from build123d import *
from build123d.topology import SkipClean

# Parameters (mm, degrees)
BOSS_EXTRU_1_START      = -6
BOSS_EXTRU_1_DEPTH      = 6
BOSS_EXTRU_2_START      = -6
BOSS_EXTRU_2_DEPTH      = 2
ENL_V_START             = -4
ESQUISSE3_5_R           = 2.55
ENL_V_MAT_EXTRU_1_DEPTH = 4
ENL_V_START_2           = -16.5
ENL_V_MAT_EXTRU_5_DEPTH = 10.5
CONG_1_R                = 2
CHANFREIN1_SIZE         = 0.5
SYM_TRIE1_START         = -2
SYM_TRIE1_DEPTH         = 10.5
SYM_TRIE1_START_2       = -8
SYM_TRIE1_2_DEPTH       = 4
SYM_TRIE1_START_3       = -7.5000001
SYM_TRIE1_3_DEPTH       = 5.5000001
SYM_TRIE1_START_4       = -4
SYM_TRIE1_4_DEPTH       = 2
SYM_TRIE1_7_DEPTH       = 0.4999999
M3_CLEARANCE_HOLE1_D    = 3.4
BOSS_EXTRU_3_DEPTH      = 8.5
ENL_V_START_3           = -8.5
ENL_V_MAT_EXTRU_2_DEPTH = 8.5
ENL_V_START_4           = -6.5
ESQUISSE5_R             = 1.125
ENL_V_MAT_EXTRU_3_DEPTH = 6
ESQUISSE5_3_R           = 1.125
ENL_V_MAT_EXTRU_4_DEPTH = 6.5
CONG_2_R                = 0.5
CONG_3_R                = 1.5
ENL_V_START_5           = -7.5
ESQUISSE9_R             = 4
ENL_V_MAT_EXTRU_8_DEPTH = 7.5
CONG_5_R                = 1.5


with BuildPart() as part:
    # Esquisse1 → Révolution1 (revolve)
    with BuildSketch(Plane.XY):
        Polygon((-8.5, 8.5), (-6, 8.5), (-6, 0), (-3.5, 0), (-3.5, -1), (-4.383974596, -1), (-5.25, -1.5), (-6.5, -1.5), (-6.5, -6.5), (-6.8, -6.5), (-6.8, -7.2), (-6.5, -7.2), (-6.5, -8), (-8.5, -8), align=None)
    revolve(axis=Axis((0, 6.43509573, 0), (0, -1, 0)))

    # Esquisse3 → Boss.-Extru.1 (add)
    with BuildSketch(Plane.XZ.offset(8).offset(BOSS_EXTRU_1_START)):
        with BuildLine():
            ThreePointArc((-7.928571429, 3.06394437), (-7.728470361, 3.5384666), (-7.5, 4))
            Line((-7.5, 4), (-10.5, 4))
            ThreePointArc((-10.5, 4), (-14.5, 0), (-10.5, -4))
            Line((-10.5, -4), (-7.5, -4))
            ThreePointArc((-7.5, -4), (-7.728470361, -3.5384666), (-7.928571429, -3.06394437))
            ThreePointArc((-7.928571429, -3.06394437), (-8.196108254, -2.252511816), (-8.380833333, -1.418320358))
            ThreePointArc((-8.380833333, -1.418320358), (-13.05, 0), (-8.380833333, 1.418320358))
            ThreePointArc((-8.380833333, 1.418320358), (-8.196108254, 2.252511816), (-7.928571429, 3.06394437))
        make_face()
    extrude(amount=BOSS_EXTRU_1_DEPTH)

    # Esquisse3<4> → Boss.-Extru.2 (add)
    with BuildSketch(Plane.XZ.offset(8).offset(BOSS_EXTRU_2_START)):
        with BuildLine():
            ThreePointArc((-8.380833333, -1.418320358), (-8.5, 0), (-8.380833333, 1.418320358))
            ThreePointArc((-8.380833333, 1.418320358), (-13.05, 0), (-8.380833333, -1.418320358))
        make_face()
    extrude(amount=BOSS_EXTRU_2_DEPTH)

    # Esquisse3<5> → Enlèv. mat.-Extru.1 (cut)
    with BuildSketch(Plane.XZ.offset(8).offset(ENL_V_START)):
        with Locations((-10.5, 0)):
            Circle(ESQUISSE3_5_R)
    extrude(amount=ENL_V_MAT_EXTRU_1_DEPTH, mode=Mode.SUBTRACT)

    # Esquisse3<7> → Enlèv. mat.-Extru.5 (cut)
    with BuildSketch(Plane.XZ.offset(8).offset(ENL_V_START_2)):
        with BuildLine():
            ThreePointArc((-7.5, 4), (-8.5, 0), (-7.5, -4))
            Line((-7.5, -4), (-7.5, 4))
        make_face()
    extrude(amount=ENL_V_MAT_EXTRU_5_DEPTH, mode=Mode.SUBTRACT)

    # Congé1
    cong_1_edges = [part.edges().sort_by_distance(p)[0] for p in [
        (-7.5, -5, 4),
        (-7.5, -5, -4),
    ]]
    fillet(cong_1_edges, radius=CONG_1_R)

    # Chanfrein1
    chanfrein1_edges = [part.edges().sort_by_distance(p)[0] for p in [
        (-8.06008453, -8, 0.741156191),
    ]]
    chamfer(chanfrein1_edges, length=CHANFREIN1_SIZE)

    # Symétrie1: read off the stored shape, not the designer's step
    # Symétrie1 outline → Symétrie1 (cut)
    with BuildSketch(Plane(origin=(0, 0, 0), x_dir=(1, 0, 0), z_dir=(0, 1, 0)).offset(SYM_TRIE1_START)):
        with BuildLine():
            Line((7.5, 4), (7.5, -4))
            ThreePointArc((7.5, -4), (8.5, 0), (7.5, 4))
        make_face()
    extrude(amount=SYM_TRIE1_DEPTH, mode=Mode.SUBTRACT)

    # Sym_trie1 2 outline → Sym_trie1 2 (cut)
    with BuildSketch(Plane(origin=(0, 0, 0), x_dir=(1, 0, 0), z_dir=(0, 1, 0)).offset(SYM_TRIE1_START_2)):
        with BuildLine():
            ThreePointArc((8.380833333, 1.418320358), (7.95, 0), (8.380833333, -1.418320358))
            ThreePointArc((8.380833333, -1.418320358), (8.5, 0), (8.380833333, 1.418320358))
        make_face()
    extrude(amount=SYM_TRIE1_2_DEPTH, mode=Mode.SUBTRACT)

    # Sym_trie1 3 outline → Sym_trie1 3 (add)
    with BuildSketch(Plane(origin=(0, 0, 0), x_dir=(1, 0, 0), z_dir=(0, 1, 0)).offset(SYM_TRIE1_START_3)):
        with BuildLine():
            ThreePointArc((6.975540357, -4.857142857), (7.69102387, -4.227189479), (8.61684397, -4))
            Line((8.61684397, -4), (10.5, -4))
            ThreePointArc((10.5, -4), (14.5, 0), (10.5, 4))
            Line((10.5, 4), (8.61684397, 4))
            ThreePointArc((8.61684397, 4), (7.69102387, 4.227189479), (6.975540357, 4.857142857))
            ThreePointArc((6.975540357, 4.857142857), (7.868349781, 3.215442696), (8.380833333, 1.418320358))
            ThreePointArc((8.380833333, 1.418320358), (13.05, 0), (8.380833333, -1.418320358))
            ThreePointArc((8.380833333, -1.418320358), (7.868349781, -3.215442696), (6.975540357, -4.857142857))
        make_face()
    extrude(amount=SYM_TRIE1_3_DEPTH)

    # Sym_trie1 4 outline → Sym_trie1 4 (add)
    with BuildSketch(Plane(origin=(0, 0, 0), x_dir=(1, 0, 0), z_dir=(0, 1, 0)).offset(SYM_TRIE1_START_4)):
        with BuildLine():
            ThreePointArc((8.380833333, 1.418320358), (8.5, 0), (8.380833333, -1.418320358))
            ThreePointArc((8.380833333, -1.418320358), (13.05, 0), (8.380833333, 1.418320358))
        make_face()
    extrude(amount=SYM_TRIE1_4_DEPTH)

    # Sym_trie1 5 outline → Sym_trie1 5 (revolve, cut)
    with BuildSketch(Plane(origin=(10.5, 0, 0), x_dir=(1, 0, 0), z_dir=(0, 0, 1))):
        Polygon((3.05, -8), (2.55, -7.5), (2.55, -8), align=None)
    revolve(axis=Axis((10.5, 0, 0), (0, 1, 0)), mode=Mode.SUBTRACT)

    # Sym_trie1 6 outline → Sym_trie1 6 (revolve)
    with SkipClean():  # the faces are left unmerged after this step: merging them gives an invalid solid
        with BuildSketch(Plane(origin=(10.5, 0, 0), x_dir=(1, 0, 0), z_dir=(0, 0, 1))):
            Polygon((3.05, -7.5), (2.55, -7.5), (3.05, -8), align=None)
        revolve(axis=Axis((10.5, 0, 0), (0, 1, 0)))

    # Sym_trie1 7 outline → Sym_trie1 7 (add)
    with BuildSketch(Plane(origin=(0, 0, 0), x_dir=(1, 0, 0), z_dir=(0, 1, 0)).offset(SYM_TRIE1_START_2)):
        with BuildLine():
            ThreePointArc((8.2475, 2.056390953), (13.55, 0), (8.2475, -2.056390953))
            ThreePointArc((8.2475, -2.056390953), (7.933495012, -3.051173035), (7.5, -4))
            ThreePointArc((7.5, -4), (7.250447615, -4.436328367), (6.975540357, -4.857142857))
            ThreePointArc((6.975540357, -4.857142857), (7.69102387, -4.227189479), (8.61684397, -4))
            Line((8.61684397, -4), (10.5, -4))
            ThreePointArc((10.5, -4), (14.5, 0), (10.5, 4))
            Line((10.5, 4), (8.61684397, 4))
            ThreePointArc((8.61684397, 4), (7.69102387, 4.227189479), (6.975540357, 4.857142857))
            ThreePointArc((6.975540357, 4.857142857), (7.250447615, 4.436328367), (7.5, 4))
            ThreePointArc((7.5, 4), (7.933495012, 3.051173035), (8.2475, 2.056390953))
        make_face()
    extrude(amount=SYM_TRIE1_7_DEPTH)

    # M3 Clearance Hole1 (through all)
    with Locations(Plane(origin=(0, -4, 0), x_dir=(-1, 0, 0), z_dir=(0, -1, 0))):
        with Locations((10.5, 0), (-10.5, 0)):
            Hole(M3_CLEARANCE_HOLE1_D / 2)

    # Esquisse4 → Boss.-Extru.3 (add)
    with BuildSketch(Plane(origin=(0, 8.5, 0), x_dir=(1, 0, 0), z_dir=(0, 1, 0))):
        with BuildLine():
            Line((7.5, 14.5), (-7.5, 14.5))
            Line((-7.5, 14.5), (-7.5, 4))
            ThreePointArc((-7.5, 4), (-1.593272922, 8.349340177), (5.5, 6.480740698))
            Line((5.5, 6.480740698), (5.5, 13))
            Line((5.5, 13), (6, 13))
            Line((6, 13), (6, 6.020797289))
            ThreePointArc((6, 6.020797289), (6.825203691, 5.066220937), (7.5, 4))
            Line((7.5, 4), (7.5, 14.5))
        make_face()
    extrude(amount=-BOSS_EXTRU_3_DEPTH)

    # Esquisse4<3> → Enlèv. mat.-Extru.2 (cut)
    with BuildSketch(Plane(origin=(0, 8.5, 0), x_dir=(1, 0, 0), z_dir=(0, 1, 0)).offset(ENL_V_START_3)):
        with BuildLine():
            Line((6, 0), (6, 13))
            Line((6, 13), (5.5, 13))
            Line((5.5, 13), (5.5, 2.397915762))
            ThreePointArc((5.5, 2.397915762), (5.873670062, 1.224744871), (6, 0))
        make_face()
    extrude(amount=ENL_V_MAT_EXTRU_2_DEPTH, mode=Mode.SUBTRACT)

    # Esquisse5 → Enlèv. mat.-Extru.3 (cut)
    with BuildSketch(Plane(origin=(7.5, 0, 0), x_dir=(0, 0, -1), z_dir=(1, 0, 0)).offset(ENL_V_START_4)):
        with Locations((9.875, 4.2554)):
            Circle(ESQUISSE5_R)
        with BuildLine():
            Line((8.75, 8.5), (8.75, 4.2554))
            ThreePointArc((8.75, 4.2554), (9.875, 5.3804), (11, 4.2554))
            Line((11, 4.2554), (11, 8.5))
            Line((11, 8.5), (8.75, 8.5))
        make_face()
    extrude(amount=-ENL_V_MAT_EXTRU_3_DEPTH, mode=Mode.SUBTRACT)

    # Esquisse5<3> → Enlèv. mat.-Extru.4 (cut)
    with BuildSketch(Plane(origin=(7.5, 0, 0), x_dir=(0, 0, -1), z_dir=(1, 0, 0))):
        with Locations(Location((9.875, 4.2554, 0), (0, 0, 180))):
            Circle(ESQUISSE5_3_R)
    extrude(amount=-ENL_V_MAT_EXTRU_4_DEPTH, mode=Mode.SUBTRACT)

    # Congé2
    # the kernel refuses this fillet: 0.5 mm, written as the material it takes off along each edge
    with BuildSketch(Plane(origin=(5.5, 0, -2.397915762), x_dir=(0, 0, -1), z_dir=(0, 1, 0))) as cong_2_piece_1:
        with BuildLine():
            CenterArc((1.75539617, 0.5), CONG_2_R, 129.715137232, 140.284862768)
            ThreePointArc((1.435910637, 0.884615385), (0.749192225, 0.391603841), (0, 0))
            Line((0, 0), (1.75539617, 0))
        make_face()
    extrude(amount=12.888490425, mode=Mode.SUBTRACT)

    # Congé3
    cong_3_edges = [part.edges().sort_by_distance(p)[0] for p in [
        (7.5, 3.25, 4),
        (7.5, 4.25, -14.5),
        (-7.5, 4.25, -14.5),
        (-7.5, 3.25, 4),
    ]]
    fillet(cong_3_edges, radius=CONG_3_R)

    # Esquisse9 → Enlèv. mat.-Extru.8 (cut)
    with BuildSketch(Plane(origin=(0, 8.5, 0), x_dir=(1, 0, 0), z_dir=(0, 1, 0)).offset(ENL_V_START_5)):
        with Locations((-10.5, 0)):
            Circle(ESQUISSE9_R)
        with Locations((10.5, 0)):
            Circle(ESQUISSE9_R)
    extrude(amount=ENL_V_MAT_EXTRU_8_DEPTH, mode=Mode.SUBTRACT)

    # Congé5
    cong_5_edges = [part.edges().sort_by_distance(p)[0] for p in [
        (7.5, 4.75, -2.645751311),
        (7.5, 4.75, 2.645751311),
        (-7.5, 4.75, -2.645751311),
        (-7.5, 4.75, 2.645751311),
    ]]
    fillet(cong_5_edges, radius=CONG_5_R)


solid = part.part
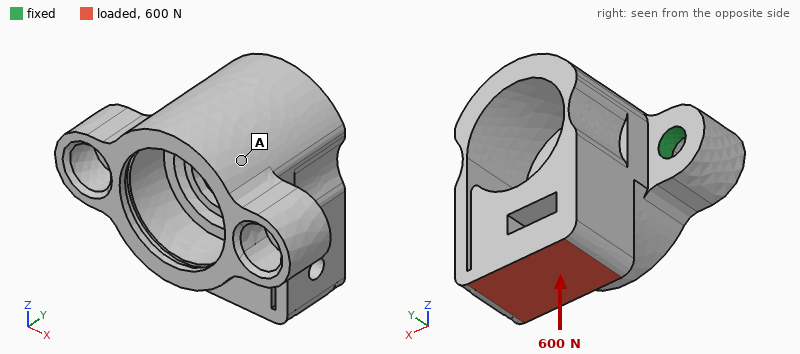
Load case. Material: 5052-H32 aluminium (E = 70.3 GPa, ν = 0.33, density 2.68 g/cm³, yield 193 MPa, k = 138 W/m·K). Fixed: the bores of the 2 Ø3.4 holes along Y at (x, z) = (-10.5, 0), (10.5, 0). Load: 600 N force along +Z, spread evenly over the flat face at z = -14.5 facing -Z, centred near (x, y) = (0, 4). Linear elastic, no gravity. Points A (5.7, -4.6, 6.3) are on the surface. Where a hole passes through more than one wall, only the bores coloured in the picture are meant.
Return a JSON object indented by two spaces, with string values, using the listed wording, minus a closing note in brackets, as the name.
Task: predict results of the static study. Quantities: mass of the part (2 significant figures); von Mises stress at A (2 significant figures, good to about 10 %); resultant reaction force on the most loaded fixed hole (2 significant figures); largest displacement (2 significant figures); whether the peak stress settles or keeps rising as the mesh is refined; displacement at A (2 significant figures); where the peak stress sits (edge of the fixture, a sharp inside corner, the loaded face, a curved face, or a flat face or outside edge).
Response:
{
  "mass of the part": "7.4 g",
  "von Mises stress at A": "27 MPa",
  "resultant reaction force on the most loaded fixed hole": "300 N",
  "largest displacement": "84 µm",
  "whether the peak stress settles or keeps rising as the mesh is refined": "keeps rising",
  "displacement at A": "21 µm",
  "where the peak stress sits": "edge of the fixture"
}
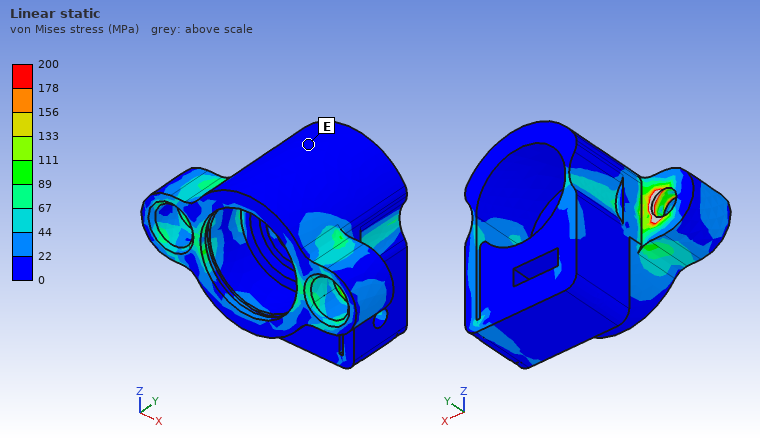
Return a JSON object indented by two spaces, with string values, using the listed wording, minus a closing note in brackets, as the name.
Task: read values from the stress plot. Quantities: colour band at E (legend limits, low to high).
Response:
{
  "colour band at E": "0 to 22 MPa"
}
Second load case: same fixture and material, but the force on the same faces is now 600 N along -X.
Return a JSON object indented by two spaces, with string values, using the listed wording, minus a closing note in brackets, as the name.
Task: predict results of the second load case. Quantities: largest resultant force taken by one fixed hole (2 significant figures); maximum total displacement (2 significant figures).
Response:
{
  "largest resultant force taken by one fixed hole": "610 N",
  "maximum total displacement": "27 µm"
}
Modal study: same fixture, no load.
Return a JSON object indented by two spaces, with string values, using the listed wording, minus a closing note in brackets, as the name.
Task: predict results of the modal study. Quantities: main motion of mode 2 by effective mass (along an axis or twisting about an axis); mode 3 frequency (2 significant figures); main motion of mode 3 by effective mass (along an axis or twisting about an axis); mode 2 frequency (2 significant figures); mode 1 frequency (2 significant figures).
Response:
{
  "main motion of mode 2 by effective mass": "along X",
  "mode 3 frequency": "21 kHz",
  "main motion of mode 3 by effective mass": "along Y",
  "mode 2 frequency": "17 kHz",
  "mode 1 frequency": "6500 Hz"
}
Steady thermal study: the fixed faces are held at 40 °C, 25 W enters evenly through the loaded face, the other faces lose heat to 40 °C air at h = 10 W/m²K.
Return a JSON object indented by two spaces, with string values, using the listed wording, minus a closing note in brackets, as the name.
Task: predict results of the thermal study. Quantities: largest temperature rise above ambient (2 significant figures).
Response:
{
  "largest temperature rise above ambient": "56 K"
}
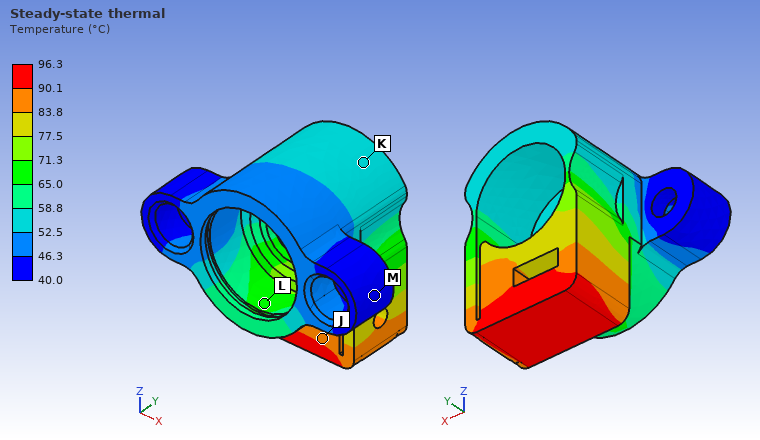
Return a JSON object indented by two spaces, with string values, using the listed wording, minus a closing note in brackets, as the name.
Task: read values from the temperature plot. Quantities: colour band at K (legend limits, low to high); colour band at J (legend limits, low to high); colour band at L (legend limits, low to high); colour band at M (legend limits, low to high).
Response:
{
  "colour band at K": "52.5 to 58.8 °C",
  "colour band at J": "83.8 to 90.1 °C",
  "colour band at L": "65.0 to 71.3 °C",
  "colour band at M": "40.0 to 46.3 °C"
}
